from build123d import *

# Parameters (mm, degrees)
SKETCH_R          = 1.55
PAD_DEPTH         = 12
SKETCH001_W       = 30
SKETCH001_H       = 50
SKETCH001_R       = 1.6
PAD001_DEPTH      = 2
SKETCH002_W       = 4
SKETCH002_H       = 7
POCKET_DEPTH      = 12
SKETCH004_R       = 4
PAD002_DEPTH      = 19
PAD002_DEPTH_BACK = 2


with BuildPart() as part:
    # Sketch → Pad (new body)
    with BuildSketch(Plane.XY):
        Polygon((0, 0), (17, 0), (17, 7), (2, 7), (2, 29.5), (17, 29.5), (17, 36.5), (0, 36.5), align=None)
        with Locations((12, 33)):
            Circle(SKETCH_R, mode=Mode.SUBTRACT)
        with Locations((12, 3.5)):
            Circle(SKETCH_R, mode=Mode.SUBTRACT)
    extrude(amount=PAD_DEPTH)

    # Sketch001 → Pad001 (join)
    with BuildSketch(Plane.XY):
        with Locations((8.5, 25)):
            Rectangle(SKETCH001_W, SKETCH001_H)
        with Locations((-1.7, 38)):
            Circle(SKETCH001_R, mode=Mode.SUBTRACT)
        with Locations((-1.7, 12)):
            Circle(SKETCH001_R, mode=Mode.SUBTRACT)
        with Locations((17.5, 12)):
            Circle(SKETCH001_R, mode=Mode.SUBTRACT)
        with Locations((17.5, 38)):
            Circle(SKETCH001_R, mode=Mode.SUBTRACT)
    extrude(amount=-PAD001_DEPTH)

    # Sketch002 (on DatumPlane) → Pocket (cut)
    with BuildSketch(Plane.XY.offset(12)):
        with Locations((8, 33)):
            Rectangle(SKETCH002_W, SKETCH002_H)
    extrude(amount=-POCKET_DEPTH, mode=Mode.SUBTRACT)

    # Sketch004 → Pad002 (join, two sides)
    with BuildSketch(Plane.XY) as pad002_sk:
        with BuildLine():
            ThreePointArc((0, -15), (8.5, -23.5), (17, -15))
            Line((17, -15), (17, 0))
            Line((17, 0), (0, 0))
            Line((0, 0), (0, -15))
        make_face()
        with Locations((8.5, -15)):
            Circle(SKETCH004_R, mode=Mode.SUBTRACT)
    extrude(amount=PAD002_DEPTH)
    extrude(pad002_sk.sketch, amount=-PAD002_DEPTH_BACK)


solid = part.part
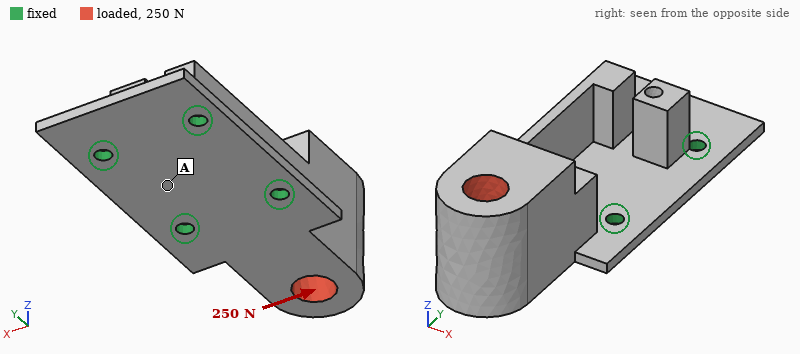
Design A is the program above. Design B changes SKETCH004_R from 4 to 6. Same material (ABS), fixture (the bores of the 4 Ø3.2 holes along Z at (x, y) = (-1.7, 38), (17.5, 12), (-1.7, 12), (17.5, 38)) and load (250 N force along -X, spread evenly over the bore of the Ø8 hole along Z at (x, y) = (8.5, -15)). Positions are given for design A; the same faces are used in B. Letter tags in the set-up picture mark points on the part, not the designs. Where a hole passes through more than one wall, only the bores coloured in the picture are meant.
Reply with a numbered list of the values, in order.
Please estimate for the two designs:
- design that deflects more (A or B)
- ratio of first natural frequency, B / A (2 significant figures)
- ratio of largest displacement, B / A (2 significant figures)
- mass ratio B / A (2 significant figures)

1. B
2. 1.2
3. 1.1
4. 0.89
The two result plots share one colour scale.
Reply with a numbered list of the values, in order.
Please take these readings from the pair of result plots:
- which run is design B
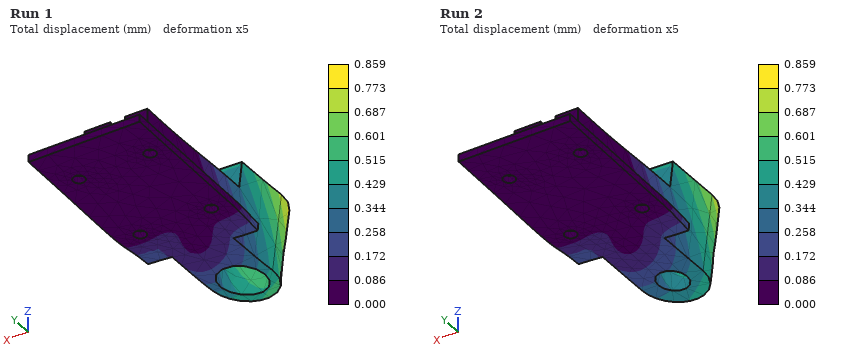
1. Run 1
